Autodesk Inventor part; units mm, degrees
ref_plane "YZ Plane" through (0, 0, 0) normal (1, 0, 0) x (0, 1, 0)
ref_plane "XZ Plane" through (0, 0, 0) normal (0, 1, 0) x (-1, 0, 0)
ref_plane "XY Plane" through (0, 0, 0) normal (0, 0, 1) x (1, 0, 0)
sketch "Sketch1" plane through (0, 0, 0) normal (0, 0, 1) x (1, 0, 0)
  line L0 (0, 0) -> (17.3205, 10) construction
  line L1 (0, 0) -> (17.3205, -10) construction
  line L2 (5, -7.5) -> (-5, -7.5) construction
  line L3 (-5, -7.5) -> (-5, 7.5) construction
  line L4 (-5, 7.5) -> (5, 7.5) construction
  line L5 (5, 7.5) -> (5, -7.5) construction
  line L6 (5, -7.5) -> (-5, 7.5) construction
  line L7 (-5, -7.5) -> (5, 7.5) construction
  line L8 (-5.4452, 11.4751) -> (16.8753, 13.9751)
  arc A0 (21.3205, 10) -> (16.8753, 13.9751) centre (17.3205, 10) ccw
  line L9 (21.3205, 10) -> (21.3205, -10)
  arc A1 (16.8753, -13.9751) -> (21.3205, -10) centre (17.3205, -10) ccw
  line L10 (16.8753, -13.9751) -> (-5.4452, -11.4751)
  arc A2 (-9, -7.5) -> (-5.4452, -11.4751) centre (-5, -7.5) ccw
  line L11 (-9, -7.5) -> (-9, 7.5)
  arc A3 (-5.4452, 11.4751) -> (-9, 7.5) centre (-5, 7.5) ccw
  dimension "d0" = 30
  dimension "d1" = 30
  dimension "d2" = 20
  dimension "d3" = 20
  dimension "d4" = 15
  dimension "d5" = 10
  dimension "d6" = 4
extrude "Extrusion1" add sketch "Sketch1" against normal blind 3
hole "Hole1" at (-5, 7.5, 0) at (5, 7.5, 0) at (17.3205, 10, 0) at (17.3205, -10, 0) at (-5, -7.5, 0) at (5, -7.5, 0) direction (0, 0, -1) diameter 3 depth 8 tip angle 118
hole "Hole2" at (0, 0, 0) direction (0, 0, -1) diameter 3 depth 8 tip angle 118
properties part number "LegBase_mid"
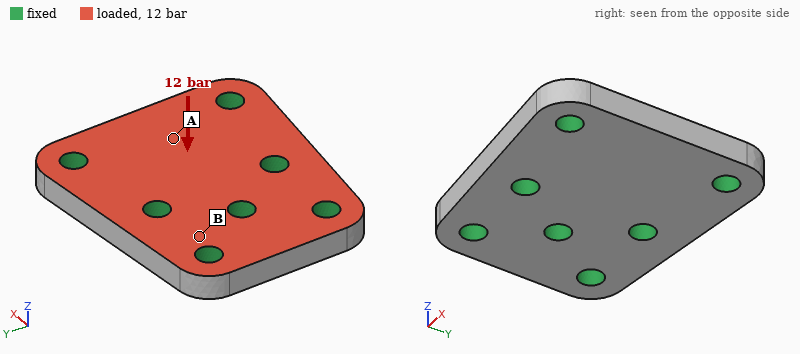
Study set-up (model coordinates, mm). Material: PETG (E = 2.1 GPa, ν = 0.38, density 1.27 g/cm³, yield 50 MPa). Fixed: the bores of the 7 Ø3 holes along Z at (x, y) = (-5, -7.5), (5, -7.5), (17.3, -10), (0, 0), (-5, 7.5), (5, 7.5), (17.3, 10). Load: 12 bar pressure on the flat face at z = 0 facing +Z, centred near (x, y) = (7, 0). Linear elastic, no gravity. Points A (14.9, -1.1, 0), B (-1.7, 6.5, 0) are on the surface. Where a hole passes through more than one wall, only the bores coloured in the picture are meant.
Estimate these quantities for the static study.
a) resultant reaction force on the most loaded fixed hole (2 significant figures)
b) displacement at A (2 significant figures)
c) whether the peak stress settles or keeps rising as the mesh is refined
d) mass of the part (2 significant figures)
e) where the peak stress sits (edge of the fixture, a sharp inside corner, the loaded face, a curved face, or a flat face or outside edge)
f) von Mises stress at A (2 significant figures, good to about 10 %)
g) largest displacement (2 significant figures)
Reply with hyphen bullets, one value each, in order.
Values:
- 150 N
- 0.088 mm
- keeps rising
- 2.7 g
- edge of the fixture
- 7.8 MPa
- 0.12 mm
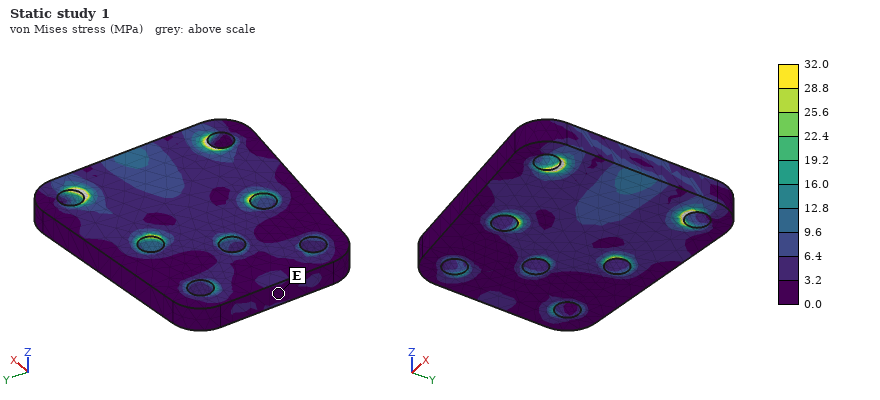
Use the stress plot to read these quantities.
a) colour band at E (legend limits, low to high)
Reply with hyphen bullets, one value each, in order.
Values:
- 0.0 to 3.2 MPa
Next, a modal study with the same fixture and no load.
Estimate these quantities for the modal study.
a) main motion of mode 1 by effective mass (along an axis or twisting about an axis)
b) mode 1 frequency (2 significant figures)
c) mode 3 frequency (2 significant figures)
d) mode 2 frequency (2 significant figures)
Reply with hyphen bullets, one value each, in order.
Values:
- along Z
- 10 kHz
- 19 kHz
- 16 kHz
